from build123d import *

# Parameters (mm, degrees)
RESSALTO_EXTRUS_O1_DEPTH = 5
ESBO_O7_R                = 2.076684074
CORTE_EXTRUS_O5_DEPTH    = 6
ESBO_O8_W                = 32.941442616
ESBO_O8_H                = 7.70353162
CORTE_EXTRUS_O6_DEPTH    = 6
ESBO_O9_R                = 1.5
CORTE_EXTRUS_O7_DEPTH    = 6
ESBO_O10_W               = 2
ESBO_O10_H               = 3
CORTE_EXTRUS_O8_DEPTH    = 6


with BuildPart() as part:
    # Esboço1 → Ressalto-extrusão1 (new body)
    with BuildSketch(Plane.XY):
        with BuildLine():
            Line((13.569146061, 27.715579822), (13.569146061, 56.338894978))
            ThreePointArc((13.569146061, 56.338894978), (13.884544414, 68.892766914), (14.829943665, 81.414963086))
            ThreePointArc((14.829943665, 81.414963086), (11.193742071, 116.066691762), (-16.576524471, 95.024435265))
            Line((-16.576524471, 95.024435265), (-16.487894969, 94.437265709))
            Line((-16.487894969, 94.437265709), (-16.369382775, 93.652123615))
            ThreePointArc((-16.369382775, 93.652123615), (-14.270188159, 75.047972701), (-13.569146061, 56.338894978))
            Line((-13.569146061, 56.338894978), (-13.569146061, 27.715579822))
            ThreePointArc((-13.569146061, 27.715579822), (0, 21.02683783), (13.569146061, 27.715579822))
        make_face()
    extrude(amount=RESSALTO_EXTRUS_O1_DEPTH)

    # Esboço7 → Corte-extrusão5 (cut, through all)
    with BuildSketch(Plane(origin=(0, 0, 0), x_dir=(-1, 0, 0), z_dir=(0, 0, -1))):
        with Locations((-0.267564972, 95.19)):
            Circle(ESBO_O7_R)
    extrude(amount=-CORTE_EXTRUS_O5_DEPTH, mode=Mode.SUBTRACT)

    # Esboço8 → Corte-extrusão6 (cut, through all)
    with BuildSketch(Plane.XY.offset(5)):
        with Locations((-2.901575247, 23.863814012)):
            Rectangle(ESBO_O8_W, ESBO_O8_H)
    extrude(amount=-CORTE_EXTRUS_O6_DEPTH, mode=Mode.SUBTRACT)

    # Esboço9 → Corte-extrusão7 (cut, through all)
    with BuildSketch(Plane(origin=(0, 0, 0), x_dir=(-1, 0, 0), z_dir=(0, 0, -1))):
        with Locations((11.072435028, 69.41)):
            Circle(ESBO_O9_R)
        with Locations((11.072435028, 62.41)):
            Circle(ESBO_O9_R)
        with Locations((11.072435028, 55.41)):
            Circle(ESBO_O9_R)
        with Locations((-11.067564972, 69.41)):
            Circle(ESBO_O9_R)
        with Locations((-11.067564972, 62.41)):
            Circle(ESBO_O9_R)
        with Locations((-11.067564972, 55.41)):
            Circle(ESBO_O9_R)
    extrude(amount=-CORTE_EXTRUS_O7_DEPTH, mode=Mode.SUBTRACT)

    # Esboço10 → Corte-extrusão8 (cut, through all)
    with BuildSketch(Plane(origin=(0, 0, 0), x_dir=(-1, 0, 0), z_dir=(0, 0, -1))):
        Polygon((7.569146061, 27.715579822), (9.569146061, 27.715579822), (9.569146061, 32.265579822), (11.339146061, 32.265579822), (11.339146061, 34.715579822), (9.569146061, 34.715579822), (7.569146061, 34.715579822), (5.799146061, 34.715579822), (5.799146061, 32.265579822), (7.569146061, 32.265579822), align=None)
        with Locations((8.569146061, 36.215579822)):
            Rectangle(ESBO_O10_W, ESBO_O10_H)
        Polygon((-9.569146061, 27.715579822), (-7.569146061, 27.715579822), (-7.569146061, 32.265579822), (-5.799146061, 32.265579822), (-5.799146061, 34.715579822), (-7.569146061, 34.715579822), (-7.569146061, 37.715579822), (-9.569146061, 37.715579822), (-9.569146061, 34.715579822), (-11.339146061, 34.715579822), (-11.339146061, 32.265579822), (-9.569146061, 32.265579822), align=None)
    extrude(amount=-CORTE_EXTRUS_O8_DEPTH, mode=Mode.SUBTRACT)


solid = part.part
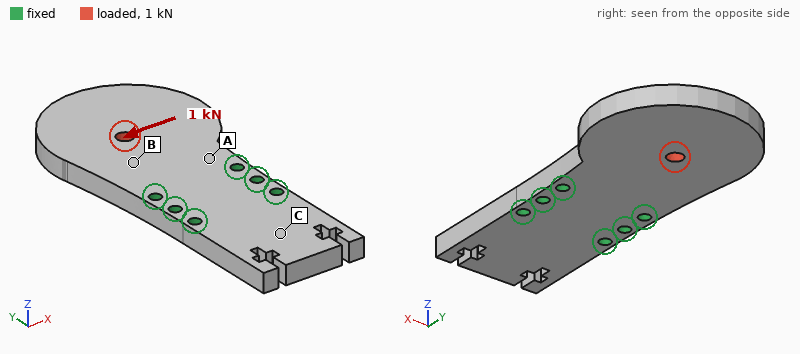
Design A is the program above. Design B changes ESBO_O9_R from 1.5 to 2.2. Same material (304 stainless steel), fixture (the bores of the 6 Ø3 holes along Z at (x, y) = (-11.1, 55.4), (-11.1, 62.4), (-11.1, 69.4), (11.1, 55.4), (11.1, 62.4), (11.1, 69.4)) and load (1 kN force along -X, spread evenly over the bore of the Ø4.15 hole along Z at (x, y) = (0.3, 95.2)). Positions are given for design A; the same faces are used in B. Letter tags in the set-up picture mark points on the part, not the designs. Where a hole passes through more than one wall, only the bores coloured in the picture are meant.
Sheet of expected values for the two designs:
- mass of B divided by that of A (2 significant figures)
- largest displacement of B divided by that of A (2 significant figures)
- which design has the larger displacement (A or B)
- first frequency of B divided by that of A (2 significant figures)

0.98
0.92
A
1.0
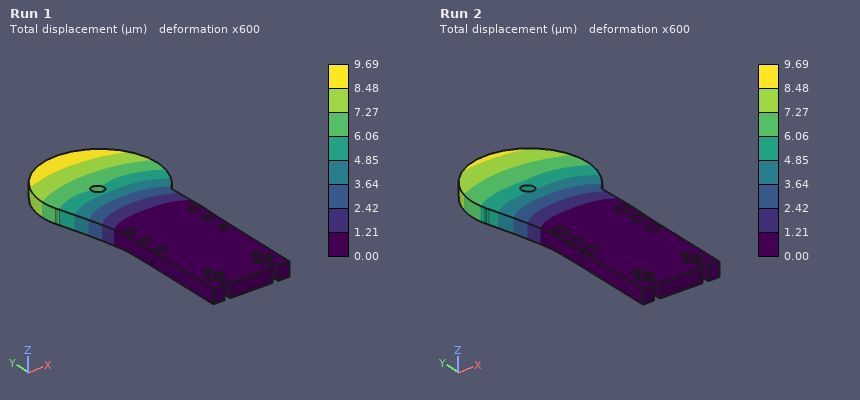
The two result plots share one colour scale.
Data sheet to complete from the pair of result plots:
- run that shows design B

Run 2
